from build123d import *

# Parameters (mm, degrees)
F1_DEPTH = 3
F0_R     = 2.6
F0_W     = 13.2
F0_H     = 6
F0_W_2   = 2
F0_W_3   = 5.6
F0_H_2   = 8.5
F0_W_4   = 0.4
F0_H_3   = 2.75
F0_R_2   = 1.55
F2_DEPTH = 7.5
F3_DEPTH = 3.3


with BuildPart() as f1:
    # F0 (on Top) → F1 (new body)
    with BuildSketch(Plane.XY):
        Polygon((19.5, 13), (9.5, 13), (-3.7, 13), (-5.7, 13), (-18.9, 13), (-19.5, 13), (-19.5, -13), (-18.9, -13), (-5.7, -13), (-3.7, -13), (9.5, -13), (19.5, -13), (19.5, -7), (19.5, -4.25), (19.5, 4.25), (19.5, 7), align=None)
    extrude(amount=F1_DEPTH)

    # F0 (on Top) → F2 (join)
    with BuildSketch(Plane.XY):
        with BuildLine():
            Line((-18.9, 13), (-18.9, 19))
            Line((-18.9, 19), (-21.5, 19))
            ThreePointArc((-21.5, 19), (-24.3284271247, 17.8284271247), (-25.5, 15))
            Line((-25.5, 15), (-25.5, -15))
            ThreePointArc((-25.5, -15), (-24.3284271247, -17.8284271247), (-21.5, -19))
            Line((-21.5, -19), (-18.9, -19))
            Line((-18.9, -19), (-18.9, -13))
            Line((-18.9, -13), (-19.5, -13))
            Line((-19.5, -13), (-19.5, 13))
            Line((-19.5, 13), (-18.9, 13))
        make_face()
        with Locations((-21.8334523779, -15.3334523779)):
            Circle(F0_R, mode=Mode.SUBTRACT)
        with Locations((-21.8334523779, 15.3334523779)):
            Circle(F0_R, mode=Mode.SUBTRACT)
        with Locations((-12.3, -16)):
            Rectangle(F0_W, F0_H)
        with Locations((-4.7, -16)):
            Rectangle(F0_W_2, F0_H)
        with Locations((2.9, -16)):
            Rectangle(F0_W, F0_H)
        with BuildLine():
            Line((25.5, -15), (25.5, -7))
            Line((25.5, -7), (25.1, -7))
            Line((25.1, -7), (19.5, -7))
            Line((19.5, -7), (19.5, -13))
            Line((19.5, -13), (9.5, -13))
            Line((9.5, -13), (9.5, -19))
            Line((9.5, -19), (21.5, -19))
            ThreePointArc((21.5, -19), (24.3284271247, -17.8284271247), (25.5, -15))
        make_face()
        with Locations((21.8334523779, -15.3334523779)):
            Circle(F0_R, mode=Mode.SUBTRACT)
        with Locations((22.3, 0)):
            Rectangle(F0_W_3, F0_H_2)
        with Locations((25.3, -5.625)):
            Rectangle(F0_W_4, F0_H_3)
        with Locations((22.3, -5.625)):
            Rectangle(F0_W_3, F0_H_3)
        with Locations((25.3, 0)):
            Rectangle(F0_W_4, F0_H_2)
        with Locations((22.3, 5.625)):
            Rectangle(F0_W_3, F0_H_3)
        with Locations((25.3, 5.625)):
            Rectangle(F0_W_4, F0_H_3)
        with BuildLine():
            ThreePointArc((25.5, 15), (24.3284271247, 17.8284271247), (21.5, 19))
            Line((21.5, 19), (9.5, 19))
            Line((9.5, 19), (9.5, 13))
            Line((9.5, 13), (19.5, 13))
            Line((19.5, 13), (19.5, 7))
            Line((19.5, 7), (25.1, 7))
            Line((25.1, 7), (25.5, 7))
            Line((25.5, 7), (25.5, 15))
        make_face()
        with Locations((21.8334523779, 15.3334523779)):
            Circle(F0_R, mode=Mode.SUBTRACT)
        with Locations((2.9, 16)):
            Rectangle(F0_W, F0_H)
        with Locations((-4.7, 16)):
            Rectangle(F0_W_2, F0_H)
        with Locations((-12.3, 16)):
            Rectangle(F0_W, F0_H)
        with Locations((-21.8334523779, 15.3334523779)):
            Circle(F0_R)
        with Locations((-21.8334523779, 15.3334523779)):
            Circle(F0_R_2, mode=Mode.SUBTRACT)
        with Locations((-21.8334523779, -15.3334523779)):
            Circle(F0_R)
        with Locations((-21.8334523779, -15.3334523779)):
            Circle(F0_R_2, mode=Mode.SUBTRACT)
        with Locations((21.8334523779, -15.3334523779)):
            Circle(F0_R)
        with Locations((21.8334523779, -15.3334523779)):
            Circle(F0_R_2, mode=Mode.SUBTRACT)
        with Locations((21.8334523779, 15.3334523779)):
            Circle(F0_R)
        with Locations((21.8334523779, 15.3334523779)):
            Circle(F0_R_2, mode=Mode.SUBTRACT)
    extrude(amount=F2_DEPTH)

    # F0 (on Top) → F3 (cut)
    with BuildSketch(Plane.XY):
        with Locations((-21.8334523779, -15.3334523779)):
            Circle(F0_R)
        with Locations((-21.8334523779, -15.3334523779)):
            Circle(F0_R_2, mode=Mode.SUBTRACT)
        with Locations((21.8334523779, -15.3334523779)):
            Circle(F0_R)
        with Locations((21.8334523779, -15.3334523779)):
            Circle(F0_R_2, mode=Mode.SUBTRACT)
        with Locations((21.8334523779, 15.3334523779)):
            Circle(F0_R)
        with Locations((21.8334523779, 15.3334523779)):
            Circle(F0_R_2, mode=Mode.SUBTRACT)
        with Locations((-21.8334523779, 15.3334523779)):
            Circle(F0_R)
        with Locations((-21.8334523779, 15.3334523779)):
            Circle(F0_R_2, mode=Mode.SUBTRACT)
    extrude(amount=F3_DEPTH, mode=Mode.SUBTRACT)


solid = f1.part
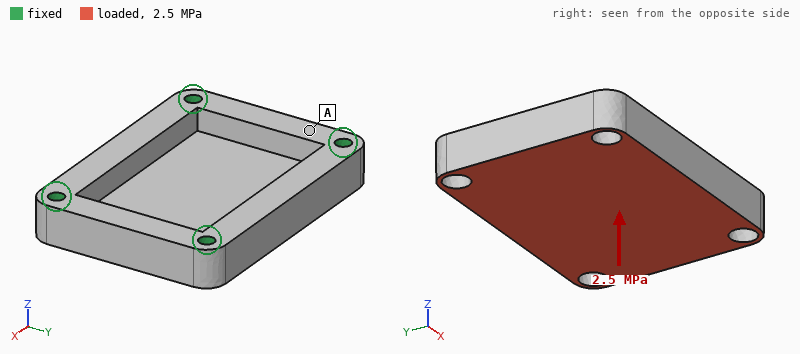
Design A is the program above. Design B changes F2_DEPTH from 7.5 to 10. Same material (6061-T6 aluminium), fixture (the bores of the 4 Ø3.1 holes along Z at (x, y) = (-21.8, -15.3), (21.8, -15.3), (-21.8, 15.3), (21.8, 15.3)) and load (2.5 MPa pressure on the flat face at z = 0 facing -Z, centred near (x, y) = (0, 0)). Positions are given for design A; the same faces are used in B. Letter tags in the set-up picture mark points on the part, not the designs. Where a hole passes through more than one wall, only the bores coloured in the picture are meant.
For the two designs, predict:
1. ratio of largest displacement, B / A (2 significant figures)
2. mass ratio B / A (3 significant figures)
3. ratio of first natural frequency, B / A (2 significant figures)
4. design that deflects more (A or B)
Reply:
0.70
1.23
1.2
A
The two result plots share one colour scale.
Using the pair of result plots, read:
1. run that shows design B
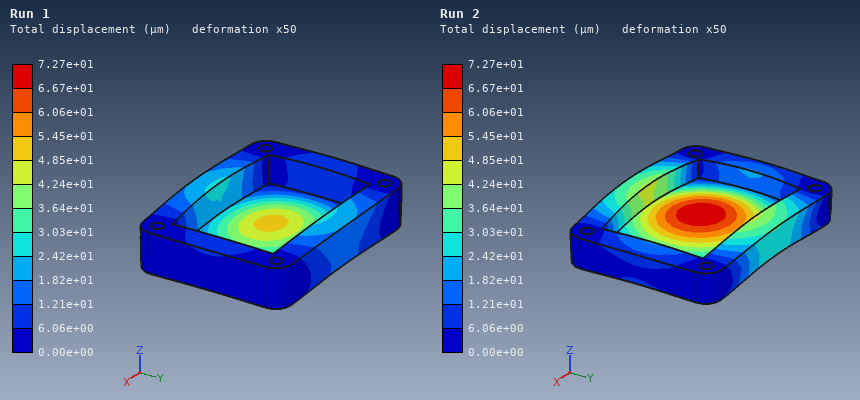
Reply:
Run 1
